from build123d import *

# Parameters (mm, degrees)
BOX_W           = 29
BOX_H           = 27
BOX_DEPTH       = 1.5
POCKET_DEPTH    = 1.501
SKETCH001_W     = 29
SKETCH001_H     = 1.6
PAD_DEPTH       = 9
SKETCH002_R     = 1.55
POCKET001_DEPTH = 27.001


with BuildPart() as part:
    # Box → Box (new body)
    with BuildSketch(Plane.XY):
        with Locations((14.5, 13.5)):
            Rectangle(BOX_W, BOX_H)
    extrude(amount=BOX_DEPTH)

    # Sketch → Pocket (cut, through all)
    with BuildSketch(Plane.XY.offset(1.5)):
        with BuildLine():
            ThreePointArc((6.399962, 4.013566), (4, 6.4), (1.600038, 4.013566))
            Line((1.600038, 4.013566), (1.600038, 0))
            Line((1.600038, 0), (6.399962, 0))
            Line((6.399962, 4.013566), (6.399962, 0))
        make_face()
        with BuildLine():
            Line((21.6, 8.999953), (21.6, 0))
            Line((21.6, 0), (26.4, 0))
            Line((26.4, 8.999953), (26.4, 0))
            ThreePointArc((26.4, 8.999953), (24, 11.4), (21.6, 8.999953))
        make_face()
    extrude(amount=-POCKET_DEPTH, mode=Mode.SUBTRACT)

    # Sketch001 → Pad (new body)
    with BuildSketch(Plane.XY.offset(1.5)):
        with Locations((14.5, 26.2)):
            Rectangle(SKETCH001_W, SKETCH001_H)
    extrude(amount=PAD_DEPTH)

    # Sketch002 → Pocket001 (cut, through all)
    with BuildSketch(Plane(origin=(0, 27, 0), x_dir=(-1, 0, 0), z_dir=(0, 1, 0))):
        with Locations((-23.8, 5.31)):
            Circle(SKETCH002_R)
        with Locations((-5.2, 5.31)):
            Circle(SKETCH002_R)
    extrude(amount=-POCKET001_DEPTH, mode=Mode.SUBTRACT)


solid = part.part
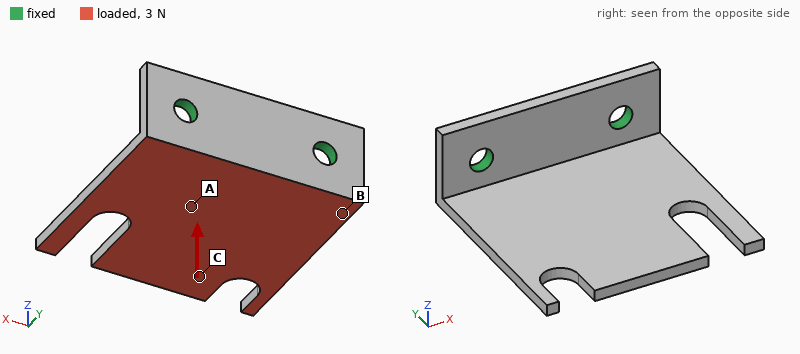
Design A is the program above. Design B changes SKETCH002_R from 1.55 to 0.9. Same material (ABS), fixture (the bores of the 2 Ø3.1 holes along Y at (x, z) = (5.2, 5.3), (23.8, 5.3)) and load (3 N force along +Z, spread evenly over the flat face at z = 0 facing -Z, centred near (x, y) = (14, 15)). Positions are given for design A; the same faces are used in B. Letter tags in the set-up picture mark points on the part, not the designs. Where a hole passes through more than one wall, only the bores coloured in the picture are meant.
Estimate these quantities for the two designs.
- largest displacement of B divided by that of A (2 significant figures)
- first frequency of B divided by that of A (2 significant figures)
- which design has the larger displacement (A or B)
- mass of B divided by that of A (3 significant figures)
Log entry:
1.1
0.95
B
1.01
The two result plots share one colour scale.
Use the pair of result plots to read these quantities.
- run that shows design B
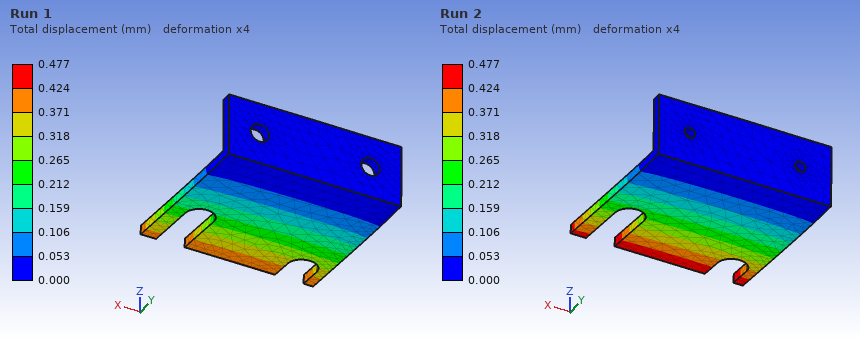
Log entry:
Run 2
